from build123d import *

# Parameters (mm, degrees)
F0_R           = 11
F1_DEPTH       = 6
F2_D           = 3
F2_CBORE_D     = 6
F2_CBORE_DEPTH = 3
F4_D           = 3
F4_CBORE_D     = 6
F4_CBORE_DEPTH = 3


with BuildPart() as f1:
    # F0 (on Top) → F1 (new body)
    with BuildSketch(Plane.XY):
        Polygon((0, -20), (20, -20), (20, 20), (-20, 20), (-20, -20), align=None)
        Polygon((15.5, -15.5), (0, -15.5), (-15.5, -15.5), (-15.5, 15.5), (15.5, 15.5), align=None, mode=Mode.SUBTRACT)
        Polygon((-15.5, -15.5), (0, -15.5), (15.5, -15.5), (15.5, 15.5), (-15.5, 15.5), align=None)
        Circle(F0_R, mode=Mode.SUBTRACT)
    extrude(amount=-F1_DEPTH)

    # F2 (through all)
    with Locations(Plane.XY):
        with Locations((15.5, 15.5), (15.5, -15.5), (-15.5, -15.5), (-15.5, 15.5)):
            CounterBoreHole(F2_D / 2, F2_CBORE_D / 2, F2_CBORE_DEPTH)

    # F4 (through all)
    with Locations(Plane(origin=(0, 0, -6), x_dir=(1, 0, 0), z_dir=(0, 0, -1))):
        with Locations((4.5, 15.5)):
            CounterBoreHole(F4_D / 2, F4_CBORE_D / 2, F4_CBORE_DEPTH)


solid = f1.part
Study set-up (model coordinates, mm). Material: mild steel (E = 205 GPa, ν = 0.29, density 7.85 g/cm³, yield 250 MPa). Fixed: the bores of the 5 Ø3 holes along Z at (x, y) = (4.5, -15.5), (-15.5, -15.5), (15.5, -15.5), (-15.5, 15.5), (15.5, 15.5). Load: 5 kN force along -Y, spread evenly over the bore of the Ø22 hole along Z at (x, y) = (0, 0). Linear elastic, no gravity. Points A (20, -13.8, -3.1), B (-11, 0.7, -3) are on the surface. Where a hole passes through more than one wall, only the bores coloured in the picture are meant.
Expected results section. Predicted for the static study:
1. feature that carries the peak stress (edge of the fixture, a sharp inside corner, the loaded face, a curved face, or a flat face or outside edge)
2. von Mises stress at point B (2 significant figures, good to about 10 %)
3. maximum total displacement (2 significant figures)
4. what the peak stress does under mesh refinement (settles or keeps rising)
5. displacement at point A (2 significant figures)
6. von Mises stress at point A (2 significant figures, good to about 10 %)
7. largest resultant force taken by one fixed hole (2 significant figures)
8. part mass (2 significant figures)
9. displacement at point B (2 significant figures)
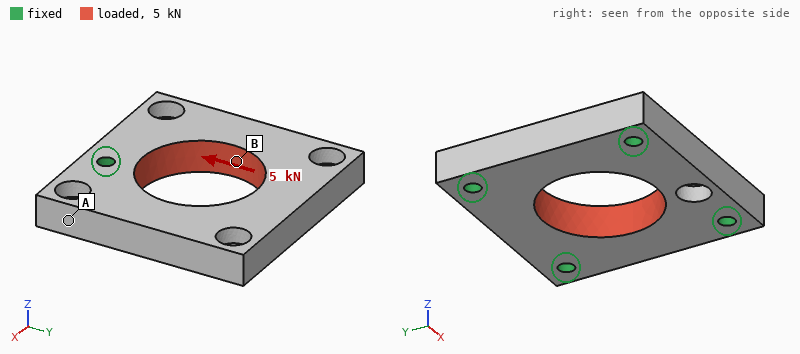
edge of the fixture
27 MPa
4.5 µm
keeps rising
0.72 µm
11 MPa
1.2 kN
53 g
1.9 µm
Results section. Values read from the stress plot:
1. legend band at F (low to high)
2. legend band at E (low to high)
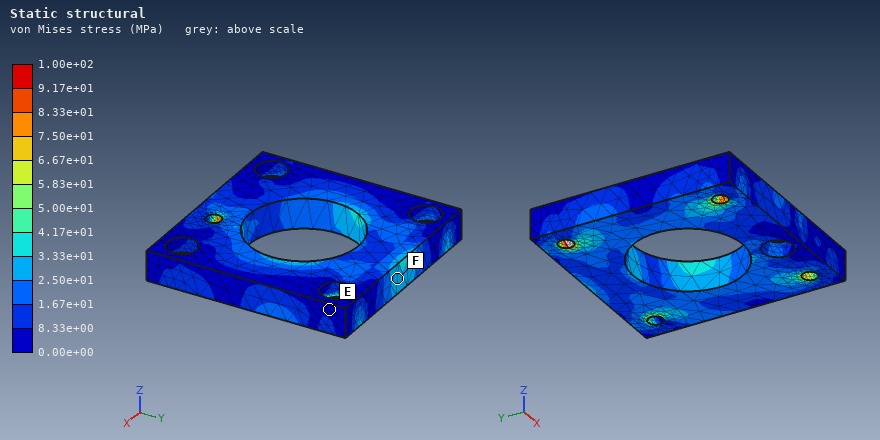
2.50e+01 to 3.33e+01 MPa
0.00e+00 to 8.33e+00 MPa
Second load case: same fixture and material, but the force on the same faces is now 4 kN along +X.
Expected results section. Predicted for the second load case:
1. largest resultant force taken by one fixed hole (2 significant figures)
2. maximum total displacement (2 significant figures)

1.0 kN
3.2 µm
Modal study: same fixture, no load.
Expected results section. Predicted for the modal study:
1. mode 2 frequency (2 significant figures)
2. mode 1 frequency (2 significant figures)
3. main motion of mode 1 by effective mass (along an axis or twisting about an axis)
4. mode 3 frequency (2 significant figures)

22 kHz
20 kHz
along Z
23 kHz
